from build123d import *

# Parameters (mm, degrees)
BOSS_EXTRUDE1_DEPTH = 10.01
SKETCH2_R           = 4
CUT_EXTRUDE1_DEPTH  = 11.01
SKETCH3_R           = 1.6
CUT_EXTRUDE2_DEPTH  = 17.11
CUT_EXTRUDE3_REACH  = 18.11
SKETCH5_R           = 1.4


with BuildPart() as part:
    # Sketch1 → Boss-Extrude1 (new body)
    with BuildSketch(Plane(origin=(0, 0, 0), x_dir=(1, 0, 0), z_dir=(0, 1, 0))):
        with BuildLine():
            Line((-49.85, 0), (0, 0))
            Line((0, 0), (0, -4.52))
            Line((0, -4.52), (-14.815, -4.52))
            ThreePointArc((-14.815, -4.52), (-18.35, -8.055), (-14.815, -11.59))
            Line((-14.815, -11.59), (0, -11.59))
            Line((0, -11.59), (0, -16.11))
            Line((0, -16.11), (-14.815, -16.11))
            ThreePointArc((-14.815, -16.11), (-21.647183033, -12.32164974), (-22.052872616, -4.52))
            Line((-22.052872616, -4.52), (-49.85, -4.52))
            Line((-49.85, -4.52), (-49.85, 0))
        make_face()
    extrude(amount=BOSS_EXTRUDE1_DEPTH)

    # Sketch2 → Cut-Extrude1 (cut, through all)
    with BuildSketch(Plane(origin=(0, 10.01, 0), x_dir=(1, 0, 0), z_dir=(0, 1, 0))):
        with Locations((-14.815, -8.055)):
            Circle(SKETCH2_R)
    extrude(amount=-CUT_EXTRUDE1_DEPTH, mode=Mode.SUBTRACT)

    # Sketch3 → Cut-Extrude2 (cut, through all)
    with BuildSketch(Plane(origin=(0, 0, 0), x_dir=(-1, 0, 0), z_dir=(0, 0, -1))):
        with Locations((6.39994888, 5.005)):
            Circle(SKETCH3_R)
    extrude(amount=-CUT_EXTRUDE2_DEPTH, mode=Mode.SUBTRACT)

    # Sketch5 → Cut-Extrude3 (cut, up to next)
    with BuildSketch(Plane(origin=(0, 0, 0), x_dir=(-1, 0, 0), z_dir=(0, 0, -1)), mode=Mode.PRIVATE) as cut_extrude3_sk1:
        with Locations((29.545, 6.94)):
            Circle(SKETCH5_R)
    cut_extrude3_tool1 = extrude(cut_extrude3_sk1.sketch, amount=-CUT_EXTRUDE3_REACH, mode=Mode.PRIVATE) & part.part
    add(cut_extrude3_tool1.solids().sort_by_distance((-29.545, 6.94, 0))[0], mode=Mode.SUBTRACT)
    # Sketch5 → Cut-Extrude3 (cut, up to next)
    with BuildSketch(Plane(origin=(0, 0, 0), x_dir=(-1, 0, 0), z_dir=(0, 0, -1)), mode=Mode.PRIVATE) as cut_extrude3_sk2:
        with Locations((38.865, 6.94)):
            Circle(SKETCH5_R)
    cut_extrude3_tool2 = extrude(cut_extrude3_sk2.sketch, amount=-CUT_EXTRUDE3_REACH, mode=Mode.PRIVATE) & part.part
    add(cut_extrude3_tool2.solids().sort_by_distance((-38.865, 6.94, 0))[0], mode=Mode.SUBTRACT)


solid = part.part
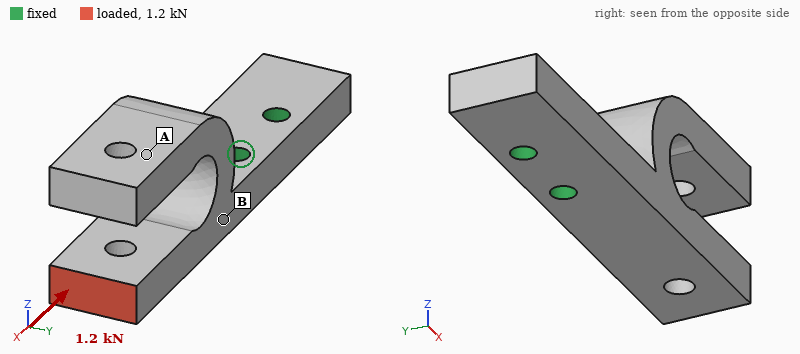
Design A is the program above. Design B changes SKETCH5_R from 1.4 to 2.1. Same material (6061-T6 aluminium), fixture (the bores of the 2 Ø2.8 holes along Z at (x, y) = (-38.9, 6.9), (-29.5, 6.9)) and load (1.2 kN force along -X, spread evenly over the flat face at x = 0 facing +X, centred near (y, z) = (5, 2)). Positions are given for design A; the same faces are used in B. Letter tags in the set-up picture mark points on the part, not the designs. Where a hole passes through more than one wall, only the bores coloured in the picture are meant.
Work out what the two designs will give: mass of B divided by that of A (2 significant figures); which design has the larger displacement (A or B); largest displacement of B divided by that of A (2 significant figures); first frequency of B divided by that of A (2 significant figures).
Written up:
0.98
A
0.90
1.1
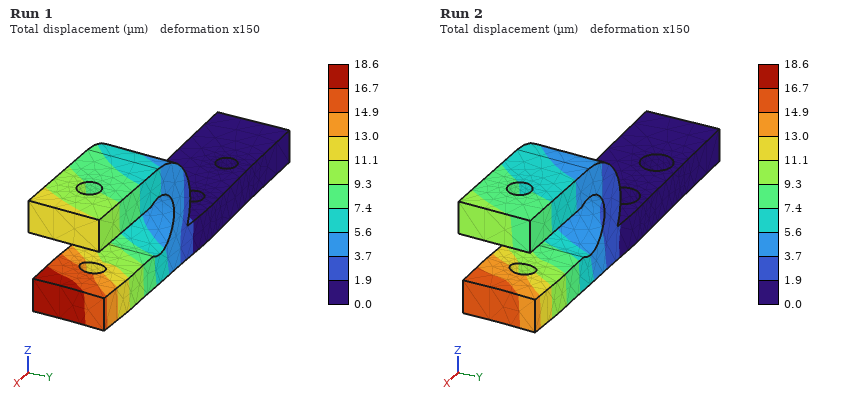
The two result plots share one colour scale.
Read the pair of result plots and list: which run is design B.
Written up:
Run 2
